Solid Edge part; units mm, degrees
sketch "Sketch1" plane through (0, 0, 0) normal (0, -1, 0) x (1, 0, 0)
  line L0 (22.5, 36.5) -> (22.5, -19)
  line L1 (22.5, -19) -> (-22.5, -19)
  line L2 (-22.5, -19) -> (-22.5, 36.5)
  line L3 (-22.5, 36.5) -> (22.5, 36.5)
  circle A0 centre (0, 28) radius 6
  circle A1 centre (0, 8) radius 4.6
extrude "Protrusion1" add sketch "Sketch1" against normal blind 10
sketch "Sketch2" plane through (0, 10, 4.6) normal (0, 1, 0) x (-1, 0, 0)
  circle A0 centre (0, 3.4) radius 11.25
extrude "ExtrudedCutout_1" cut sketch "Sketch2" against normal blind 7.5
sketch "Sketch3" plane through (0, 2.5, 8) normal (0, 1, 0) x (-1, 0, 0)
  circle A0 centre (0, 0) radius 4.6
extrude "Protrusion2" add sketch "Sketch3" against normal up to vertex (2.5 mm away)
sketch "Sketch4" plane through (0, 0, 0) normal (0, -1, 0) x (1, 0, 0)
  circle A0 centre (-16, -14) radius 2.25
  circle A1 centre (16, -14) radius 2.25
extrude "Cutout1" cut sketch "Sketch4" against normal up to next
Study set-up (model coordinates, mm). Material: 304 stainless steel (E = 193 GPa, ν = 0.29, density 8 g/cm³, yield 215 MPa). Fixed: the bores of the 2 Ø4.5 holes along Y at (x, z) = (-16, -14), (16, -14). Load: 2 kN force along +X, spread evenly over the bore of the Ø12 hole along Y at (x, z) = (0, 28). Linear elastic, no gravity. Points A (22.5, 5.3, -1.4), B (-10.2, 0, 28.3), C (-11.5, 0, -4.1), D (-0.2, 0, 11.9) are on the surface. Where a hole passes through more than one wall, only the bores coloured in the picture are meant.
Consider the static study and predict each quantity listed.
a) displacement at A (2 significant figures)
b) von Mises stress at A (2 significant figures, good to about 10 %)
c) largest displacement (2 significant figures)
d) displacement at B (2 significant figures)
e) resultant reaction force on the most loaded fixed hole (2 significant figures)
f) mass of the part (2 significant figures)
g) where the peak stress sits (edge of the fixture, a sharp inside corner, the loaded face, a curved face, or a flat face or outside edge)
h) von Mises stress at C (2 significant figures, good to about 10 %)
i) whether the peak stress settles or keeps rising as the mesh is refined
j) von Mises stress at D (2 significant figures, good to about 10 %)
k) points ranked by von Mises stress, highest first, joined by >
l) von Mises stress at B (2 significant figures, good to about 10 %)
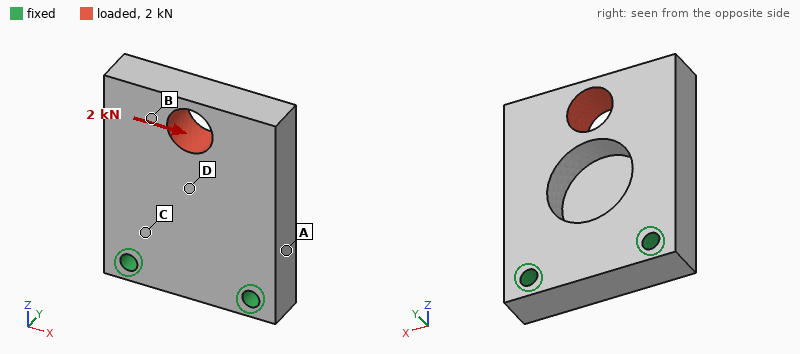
3.2 µm
27 MPa
16 µm
10 µm
2.6 kN
160 g
edge of the fixture
15 MPa
keeps rising
35 MPa
D > A > C > B
6.5 MPa
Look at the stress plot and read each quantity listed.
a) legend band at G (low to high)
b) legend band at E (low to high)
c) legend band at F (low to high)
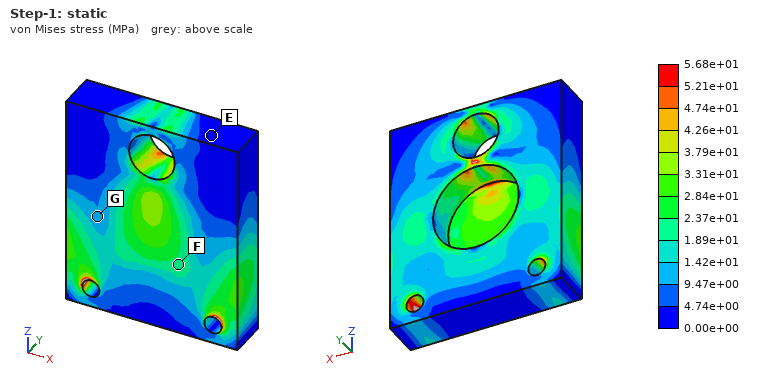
9.47e+00 to 1.42e+01 MPa
0.00e+00 to 4.74e+00 MPa
1.89e+01 to 2.37e+01 MPa
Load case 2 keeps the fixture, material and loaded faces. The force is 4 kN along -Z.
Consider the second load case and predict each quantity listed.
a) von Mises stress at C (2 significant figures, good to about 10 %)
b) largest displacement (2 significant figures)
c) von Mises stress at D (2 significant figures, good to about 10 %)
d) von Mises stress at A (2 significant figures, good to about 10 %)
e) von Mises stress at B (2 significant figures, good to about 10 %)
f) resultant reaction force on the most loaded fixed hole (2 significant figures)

11 MPa
9.9 µm
23 MPa
15 MPa
17 MPa
2.0 kN
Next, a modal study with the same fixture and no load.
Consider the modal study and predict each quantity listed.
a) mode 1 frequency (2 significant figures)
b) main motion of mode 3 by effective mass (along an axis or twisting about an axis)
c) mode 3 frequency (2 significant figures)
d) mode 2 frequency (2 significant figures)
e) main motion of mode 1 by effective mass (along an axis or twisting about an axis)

2800 Hz
along X
8500 Hz
6000 Hz
along Y
